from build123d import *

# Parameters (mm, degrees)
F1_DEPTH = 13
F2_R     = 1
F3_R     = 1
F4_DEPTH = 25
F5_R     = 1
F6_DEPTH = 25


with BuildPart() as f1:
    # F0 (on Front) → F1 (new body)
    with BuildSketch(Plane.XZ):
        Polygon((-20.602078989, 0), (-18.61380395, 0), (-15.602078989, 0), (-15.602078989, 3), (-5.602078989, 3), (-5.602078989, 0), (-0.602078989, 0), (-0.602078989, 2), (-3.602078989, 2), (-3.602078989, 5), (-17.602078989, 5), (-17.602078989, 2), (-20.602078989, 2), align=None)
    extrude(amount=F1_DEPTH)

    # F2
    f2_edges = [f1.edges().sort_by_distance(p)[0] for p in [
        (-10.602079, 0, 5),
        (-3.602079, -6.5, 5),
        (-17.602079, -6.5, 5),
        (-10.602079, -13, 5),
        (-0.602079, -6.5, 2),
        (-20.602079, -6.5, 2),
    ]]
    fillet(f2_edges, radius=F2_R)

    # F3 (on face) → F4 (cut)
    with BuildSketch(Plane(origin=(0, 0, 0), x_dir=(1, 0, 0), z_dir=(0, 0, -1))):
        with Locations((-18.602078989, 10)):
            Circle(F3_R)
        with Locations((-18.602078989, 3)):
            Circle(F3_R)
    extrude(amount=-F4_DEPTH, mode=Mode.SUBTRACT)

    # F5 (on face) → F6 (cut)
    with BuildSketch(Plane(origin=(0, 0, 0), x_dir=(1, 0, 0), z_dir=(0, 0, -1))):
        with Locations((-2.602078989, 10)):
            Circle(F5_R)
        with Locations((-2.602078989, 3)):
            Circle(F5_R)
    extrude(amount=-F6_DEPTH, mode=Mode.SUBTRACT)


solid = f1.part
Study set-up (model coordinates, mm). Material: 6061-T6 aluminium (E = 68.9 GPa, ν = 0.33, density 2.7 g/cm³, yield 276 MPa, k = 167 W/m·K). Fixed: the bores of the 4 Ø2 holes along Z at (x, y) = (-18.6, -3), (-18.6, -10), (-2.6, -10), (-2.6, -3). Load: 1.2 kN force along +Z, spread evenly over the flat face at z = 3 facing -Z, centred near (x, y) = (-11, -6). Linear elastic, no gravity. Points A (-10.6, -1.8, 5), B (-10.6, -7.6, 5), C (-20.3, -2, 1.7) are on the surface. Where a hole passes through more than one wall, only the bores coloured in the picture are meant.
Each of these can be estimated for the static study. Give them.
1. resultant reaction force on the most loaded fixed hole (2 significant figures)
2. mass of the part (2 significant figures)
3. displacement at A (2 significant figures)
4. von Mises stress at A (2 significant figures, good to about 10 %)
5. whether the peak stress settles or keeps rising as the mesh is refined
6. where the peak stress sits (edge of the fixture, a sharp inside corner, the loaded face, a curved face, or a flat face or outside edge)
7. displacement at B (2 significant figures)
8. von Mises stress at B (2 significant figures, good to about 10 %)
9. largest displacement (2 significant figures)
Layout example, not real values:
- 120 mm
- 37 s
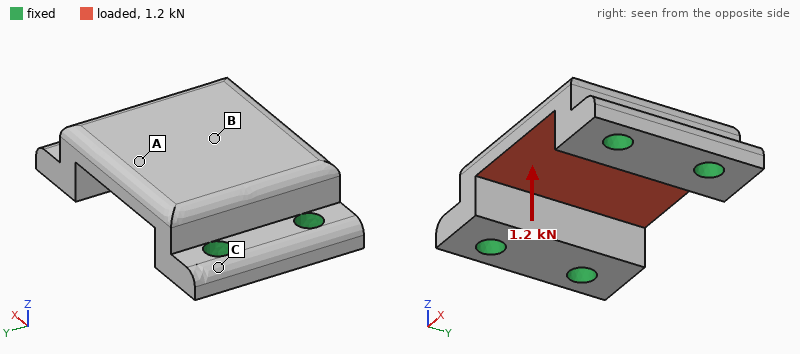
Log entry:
- 430 N
- 1.7 g
- 19 µm
- 120 MPa
- keeps rising
- edge of the fixture
- 17 µm
- 110 MPa
- 21 µm
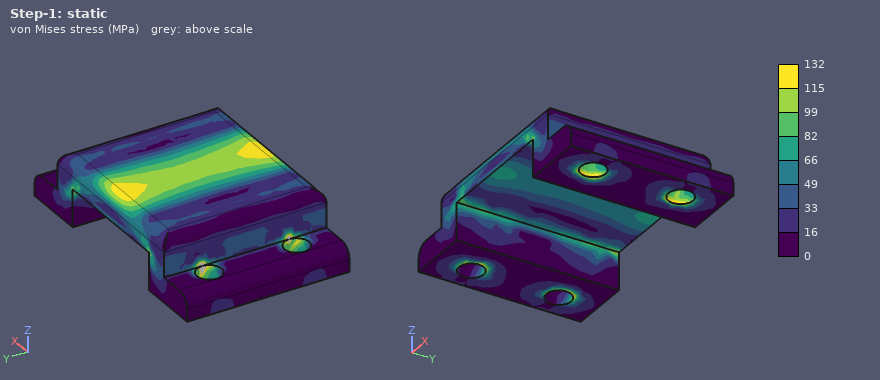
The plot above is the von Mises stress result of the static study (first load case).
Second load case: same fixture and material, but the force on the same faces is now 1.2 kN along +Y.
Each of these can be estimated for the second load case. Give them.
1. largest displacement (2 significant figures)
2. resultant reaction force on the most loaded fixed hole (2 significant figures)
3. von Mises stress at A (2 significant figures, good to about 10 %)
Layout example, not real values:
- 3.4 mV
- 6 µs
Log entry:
- 11 µm
- 350 N
- 45 MPa
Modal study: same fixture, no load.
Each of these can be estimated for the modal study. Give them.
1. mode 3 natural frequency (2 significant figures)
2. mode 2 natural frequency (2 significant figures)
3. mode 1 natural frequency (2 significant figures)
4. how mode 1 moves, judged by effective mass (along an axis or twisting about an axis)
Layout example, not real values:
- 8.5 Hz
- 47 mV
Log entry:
- 58 kHz
- 57 kHz
- 53 kHz
- along Z
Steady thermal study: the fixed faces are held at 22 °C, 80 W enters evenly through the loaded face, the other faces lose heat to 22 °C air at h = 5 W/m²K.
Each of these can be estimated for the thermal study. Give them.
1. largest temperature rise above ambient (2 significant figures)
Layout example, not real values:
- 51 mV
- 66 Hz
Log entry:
- 62 K
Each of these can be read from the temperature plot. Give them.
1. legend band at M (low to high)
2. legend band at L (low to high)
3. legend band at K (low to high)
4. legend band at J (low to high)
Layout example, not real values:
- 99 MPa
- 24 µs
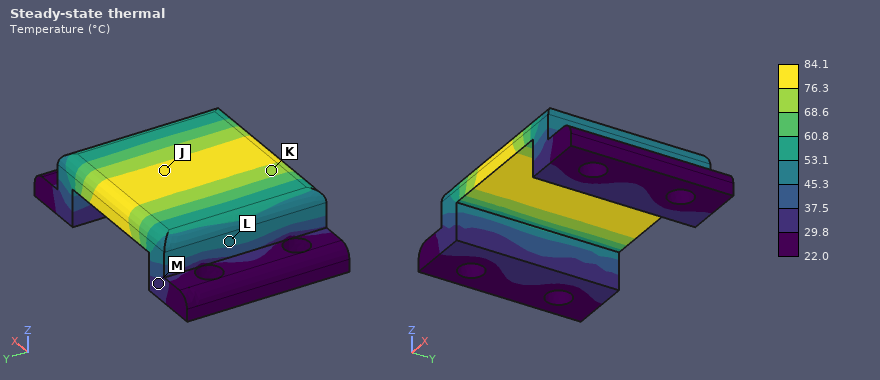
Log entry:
- 29.8 to 37.5 °C
- 45.3 to 53.1 °C
- 68.6 to 76.3 °C
- 76.3 to 84.1 °C
